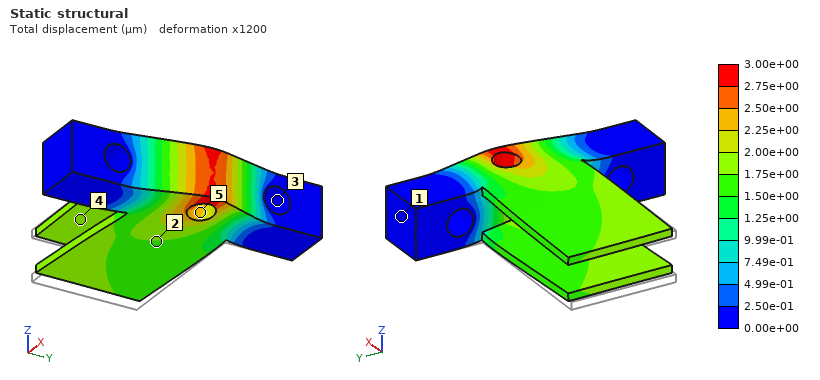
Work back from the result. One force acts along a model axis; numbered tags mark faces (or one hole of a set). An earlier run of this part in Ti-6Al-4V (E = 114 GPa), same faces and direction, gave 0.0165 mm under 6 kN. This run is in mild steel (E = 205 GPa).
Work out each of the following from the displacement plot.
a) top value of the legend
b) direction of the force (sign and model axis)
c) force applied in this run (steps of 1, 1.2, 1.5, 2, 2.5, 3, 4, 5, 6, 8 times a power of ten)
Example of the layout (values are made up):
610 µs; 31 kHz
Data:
3.00e+00 µm; +X; 2 kN
